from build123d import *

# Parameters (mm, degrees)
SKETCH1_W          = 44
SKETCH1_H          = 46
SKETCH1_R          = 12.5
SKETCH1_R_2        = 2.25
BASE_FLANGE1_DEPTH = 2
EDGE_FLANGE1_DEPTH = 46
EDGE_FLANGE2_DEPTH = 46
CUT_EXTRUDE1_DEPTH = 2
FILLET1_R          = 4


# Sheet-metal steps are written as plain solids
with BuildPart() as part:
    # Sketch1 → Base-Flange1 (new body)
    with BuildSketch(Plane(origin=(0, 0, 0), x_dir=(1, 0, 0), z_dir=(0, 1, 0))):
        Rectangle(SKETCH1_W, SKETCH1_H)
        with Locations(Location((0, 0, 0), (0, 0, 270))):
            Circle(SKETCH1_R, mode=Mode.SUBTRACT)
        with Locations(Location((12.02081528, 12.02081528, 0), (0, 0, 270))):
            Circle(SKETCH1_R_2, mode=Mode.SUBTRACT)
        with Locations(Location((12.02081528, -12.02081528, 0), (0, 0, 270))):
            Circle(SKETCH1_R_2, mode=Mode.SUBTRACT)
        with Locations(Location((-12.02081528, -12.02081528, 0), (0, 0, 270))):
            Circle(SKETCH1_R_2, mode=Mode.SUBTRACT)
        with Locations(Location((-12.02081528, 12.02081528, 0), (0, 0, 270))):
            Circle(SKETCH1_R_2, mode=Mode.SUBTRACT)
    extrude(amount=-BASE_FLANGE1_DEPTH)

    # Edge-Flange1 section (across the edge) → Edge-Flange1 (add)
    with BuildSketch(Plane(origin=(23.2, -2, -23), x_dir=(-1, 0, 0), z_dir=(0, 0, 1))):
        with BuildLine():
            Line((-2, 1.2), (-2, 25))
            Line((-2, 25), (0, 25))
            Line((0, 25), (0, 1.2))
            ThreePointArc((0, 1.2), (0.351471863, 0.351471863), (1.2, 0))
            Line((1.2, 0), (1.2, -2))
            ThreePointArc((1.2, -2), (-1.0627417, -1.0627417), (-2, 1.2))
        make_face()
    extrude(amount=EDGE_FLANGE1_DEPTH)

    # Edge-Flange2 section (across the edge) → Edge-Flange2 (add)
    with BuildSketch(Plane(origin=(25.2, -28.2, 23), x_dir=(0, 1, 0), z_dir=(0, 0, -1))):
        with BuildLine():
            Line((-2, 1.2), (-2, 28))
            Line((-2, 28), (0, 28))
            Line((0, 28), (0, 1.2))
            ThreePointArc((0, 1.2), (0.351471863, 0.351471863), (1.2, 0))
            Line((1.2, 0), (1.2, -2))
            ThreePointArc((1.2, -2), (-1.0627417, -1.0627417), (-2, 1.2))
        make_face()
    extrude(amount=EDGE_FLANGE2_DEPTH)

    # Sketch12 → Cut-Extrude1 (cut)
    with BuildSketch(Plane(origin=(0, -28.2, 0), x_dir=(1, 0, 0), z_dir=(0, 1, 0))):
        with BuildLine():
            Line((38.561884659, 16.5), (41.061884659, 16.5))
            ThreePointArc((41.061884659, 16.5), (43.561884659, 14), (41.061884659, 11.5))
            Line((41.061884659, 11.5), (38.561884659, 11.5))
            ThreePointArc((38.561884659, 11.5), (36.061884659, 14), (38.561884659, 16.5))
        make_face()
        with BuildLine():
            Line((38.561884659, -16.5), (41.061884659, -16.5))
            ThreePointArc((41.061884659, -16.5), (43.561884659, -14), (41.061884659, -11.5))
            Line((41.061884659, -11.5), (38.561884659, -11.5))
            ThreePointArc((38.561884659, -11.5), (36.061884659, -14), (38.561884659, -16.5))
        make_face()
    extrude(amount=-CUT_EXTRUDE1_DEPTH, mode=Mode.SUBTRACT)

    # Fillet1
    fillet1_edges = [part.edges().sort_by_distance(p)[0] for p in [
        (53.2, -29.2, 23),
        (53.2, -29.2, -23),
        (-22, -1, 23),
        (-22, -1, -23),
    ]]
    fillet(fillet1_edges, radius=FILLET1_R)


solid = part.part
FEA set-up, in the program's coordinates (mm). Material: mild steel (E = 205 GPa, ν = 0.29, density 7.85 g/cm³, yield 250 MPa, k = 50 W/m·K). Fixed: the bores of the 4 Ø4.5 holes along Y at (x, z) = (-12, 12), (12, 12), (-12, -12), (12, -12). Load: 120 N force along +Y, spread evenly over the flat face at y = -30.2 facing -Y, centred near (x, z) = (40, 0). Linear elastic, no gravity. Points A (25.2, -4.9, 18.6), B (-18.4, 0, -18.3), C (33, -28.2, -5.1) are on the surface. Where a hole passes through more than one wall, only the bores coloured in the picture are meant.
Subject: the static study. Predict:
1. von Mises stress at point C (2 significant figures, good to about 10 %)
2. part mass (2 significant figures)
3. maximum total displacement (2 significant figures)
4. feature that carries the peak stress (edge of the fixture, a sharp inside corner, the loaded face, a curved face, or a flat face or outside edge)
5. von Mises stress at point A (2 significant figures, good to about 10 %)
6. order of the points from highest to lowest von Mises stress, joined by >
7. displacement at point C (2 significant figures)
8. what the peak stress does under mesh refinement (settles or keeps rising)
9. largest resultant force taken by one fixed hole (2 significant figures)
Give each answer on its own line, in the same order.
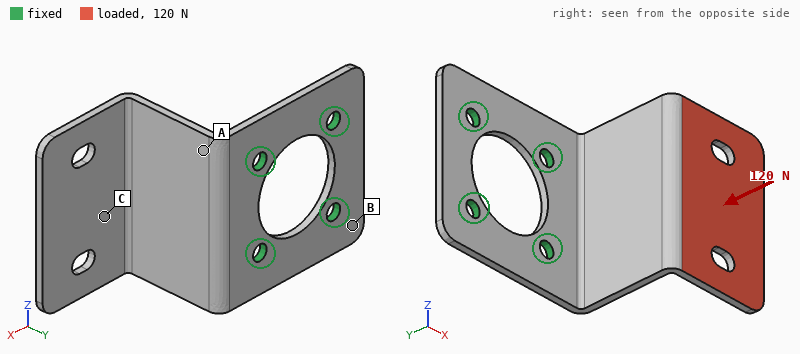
29 MPa
63 g
0.51 mm
edge of the fixture
54 MPa
A > C > B
0.27 mm
keeps rising
66 N
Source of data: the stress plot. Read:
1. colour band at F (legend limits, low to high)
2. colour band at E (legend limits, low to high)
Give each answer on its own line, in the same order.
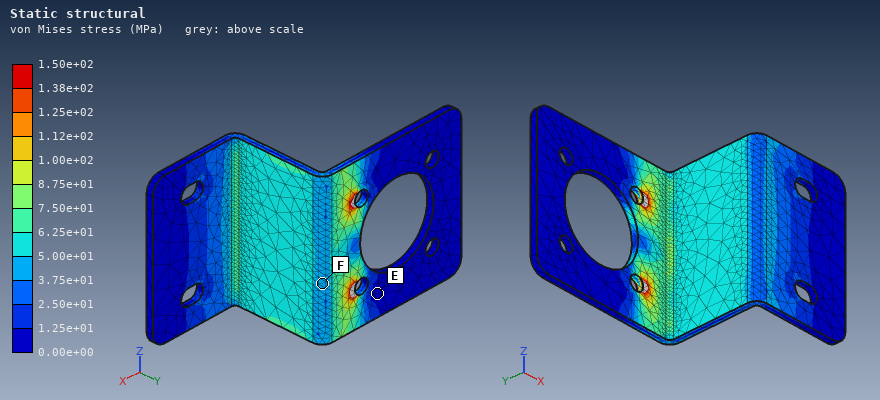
3.75e+01 to 5.00e+01 MPa
0.00e+00 to 1.25e+01 MPa
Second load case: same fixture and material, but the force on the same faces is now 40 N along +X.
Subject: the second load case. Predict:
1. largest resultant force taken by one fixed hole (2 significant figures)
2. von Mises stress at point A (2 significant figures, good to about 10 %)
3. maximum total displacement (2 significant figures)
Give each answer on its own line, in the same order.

22 N
28 MPa
0.18 mm
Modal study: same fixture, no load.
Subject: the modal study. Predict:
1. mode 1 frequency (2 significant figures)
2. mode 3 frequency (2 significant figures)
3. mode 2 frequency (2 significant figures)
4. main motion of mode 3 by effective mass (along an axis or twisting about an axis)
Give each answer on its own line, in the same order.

500 Hz
1800 Hz
1200 Hz
along X
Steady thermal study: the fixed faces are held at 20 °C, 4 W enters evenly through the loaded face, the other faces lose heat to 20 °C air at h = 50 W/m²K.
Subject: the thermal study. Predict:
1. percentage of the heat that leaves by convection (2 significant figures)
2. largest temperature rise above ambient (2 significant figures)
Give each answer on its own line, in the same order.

70 %
23 K
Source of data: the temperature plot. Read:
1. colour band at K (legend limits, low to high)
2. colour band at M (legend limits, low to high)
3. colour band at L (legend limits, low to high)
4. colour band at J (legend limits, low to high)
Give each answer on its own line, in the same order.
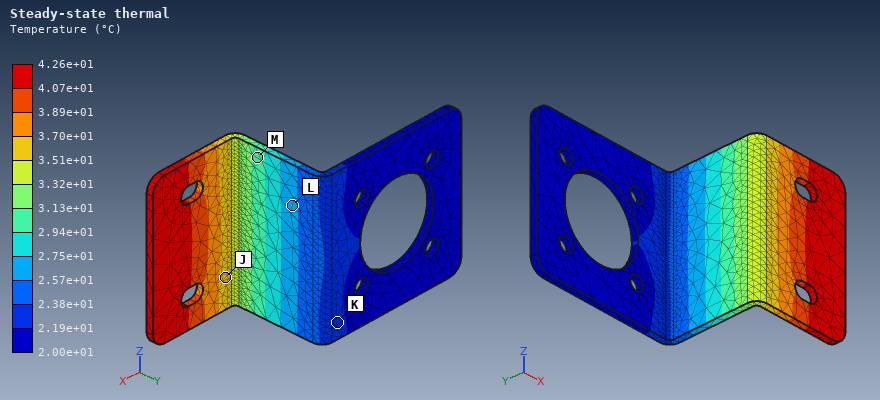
2.19e+01 to 2.38e+01 °C
2.94e+01 to 3.13e+01 °C
2.57e+01 to 2.75e+01 °C
3.51e+01 to 3.70e+01 °C
